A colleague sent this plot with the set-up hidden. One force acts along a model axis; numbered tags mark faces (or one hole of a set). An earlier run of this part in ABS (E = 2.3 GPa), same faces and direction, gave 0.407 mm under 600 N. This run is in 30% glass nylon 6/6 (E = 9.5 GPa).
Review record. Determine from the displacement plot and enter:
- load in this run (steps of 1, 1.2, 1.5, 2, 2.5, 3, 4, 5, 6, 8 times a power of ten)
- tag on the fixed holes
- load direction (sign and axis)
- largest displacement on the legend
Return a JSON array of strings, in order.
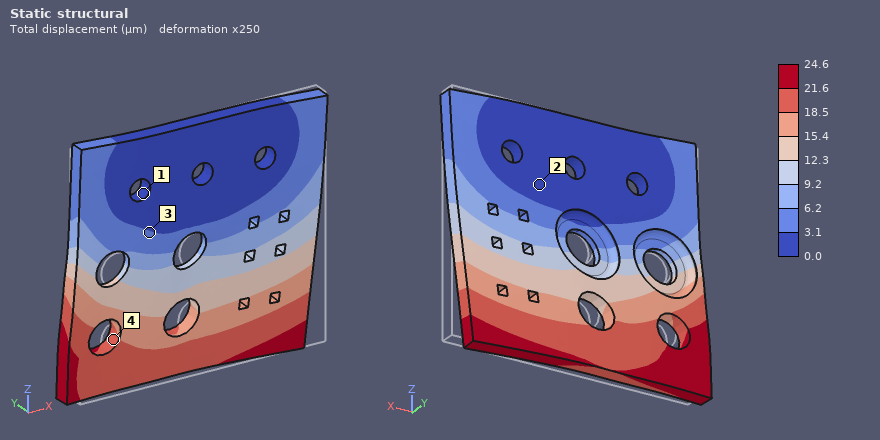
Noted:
["150 N", "1", "-X", "24.6 µm"]
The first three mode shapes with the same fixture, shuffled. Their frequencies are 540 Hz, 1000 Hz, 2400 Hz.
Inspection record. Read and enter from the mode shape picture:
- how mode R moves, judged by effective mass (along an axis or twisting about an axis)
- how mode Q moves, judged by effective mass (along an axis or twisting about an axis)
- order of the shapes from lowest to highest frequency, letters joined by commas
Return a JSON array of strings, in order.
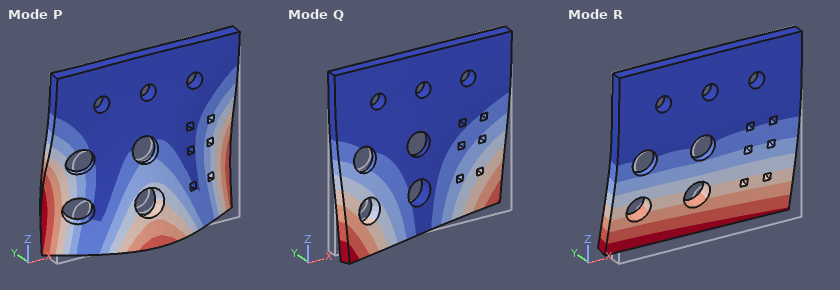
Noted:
["along Y", "twisting about Z", "R, Q, P"]
